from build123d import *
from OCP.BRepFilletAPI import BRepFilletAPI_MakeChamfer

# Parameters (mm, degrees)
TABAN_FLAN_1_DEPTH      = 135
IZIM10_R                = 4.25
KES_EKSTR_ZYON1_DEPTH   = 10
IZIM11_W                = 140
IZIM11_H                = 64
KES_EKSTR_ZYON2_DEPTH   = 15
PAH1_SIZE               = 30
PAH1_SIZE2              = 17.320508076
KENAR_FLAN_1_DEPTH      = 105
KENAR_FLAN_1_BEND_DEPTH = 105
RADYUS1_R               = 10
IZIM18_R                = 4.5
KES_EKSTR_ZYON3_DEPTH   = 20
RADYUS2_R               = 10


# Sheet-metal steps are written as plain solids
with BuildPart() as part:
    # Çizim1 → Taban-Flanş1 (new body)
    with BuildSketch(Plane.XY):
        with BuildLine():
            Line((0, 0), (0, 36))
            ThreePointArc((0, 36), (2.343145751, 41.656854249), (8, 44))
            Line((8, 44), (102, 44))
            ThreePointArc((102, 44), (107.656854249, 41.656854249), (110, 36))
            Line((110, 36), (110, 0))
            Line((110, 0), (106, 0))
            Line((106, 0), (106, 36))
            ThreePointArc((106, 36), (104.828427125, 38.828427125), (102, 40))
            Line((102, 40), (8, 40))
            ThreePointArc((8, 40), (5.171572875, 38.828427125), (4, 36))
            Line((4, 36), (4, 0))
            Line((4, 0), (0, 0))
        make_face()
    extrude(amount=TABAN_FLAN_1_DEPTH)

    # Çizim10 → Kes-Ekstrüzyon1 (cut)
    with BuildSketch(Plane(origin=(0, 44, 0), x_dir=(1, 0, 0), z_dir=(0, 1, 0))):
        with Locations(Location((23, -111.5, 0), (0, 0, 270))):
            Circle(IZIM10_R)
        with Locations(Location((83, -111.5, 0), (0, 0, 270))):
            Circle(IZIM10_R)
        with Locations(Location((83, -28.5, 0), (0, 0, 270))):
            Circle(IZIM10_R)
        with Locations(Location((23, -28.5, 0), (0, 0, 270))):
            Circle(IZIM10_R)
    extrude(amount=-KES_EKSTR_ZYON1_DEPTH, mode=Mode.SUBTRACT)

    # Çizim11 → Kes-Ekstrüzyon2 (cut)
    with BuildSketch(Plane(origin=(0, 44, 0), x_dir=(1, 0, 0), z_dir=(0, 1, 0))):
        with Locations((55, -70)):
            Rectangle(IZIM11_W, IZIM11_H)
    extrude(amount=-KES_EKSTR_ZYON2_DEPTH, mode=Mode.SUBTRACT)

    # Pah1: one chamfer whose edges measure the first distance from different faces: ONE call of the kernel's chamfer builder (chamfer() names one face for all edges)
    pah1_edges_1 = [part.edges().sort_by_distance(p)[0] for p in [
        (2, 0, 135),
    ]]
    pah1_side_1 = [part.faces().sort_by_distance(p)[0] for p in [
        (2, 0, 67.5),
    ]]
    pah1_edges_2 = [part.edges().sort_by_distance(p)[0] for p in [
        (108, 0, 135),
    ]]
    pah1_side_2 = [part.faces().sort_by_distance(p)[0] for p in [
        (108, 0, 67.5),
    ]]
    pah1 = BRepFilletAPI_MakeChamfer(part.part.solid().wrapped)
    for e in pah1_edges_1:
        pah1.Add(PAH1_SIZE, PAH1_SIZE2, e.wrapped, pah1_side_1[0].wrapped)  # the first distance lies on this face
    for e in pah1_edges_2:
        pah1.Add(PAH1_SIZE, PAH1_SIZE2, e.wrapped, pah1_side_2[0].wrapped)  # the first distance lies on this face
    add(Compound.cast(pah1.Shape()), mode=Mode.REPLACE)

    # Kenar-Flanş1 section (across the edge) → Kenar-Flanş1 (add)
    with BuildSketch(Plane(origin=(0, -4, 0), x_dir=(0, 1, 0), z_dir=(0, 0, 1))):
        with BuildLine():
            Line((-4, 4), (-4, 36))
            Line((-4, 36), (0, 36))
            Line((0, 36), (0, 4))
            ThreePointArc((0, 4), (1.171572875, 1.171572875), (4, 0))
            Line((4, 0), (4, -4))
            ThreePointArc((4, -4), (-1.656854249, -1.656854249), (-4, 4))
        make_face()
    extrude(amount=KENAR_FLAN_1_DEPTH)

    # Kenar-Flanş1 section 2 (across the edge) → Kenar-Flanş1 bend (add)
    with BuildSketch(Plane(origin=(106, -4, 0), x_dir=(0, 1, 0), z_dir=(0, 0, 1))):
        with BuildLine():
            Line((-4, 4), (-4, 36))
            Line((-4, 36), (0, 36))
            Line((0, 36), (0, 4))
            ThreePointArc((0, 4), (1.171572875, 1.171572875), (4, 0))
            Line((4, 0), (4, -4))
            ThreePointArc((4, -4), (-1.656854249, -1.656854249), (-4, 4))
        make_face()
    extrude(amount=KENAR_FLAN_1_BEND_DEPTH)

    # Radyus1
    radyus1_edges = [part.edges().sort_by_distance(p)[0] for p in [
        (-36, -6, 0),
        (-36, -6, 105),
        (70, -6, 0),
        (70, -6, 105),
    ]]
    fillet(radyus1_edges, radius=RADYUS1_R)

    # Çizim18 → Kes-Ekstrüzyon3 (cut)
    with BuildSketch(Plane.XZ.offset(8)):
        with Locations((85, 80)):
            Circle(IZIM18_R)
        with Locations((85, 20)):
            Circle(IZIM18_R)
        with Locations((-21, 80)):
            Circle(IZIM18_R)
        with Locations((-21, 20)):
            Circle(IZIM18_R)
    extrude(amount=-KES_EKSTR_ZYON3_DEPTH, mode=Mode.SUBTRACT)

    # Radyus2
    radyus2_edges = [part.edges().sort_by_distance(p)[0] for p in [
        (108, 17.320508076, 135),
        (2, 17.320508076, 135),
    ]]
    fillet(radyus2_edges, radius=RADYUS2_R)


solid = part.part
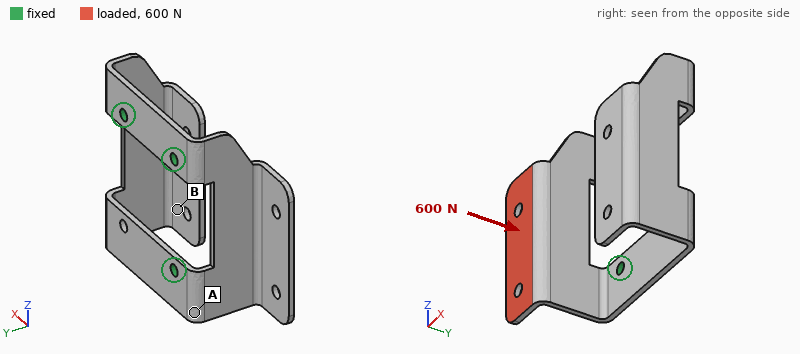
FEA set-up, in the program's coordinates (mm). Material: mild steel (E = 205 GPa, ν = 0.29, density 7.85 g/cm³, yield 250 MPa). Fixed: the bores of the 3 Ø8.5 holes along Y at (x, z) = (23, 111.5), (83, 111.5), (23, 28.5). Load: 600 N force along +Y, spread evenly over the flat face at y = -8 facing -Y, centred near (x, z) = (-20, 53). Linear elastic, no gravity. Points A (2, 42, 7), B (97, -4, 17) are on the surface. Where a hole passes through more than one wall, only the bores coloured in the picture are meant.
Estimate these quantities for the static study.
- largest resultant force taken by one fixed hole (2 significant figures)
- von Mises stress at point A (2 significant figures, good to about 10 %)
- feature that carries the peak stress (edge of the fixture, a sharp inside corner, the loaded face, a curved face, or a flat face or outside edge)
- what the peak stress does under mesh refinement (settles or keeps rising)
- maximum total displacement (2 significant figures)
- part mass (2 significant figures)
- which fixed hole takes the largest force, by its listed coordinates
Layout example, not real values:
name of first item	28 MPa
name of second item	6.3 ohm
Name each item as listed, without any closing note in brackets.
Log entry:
largest resultant force taken by one fixed hole	420 N
von Mises stress at point A	62 MPa
feature that carries the peak stress	edge of the fixture
what the peak stress does under mesh refinement	keeps rising
maximum total displacement	0.68 mm
part mass	770 g
which fixed hole takes the largest force, by its listed coordinates	(23, 28.5)
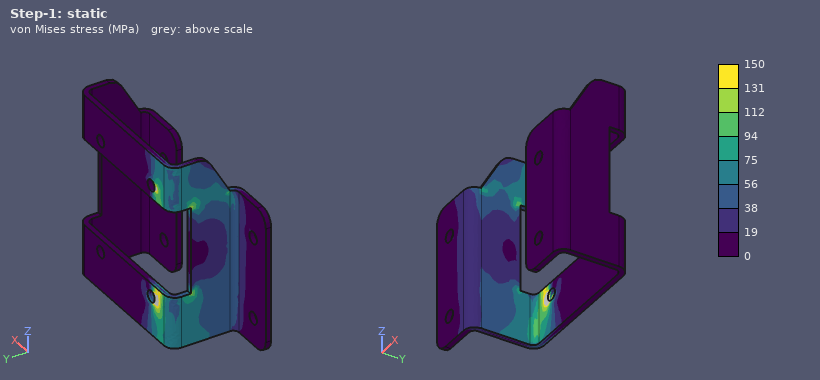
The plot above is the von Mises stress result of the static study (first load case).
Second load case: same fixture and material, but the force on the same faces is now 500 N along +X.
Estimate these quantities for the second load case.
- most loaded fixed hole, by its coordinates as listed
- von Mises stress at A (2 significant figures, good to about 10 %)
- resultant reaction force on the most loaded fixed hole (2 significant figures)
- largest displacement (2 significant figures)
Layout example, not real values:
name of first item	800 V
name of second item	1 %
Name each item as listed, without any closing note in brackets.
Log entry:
most loaded fixed hole, by its coordinates as listed	(23, 28.5)
von Mises stress at A	98 MPa
resultant reaction force on the most loaded fixed hole	310 N
largest displacement	0.81 mm
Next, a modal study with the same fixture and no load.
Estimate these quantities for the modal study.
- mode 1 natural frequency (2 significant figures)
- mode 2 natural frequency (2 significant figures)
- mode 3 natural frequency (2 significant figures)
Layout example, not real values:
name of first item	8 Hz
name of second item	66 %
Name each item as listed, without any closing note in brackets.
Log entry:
mode 1 natural frequency	250 Hz
mode 2 natural frequency	350 Hz
mode 3 natural frequency	380 Hz
